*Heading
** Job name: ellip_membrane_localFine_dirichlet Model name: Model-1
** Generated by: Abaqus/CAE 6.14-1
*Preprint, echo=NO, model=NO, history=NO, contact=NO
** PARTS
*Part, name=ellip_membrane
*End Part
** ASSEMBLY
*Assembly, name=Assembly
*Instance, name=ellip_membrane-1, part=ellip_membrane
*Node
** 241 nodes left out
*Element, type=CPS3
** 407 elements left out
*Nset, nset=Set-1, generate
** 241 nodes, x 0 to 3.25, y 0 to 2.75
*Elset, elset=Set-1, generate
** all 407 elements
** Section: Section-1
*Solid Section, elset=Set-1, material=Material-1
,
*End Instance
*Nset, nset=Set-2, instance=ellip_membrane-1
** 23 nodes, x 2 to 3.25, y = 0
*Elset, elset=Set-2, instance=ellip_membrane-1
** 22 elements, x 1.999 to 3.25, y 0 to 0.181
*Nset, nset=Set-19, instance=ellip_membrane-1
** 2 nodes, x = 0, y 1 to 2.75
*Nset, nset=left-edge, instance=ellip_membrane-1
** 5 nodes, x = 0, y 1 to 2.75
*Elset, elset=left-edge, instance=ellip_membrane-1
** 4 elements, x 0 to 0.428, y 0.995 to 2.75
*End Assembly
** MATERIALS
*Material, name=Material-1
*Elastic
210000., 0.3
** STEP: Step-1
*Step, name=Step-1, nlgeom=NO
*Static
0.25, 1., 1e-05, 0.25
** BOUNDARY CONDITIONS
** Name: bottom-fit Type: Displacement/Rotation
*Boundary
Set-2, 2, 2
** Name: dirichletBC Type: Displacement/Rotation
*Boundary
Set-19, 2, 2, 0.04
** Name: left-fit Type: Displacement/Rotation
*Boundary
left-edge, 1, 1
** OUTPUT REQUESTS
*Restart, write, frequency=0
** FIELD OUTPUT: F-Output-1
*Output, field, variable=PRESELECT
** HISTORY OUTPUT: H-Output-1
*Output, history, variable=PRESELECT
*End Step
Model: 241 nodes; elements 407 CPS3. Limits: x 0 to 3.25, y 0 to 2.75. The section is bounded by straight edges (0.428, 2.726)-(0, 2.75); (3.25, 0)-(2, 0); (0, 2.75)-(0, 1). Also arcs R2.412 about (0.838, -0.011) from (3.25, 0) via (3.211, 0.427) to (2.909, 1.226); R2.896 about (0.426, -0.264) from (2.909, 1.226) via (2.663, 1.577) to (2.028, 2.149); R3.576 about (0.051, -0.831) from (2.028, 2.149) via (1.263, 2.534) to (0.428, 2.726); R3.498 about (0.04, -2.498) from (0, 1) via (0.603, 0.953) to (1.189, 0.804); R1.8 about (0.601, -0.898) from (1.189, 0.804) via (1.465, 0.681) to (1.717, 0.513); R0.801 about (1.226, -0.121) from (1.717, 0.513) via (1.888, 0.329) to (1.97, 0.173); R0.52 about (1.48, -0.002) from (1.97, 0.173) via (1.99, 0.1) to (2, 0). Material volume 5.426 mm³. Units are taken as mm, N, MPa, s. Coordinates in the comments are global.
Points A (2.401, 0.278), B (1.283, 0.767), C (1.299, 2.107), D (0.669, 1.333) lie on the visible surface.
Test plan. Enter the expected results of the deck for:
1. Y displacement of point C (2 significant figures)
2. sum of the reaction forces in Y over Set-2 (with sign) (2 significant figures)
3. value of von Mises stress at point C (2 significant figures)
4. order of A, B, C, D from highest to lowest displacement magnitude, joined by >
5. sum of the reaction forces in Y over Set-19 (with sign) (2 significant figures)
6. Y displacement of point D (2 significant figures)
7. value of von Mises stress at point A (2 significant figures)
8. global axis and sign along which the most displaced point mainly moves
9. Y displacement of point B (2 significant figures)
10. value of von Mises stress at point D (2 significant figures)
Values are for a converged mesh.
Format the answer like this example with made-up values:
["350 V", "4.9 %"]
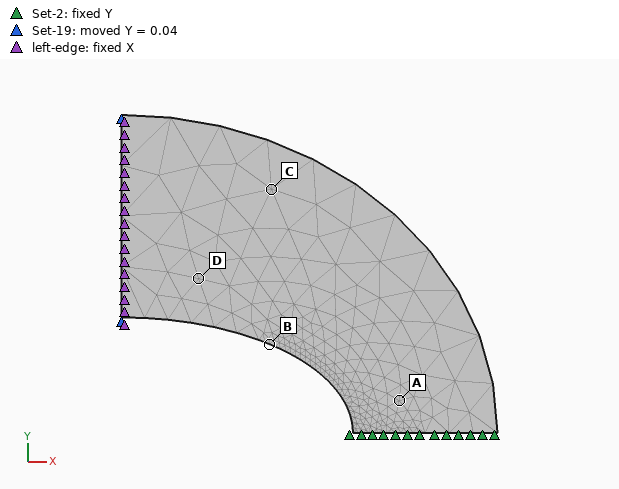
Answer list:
["0.022 mm", "-660 N", "850 MPa", "D > B > C > A", "660 N", "0.030 mm", "740 MPa", "+Y", "0.020 mm", "1000 MPa"]
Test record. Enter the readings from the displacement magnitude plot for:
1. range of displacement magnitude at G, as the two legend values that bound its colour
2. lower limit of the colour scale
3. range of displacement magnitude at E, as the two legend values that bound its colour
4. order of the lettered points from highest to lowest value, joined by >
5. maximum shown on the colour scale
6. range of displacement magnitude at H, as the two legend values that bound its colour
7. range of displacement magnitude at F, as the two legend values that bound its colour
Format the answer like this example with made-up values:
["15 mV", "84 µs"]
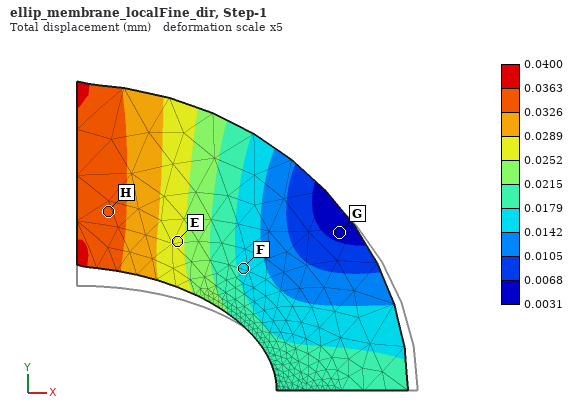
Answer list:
["0.0031 to 0.0068 mm", "0.0031 mm", "0.0252 to 0.0289 mm", "H > E > F > G", "0.0400 mm", "0.0326 to 0.0363 mm", "0.0142 to 0.0179 mm"]
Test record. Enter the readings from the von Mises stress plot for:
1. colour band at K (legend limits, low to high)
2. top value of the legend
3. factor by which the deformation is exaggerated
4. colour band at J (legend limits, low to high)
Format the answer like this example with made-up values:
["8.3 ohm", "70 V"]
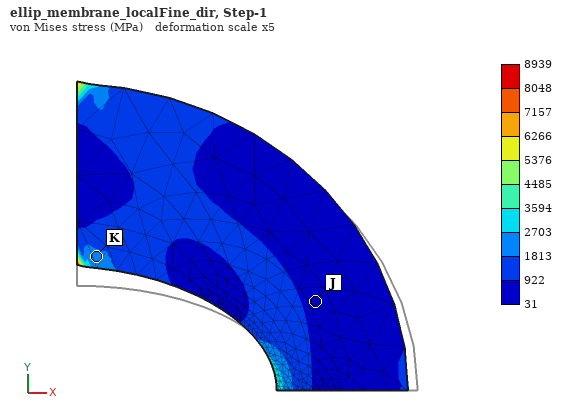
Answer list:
["1813 to 2703 MPa", "8939 MPa", "5", "31 to 922 MPa"]
